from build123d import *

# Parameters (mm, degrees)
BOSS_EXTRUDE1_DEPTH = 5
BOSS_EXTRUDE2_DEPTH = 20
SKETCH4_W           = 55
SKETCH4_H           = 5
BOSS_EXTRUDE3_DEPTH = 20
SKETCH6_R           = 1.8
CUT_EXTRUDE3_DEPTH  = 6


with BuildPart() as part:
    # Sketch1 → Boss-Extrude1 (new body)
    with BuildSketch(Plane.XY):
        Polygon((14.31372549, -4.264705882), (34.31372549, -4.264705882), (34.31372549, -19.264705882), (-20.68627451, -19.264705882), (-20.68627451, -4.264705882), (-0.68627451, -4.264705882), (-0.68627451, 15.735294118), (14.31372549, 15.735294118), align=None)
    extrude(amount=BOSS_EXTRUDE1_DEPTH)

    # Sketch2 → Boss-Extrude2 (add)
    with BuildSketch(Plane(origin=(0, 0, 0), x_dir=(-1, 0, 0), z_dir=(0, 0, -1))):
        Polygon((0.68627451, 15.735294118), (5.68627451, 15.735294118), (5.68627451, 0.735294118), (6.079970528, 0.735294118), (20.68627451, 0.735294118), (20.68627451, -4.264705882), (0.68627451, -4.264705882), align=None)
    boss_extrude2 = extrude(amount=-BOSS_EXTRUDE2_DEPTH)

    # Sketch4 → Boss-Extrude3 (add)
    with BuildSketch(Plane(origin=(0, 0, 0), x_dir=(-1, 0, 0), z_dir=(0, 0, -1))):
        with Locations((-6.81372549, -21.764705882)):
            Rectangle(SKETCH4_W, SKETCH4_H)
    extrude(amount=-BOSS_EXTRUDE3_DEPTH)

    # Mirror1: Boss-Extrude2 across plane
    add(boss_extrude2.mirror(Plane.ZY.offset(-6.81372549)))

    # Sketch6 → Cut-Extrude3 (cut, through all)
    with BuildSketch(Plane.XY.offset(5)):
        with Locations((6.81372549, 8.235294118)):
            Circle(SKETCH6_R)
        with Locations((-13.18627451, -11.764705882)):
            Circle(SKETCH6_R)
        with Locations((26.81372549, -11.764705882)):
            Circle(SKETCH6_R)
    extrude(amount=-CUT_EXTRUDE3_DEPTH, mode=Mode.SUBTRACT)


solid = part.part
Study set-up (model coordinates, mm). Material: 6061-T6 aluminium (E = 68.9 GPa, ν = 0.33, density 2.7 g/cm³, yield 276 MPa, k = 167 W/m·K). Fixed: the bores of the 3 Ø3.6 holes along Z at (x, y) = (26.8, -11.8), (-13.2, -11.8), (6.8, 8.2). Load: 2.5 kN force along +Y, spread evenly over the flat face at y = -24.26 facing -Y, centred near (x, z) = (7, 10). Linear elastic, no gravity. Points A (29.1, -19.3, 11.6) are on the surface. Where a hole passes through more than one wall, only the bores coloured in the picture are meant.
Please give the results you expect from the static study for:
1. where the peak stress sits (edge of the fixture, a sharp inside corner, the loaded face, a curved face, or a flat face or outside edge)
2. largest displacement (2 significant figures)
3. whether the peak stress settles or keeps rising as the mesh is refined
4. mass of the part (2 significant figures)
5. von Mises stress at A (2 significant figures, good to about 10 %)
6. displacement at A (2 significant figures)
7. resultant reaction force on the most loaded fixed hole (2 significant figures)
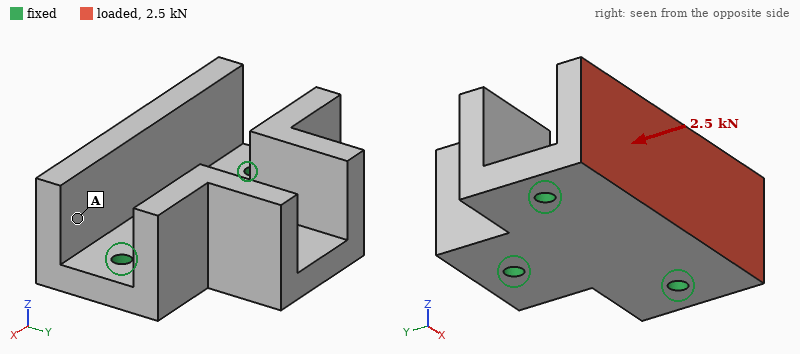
edge of the fixture
0.12 mm
keeps rising
49 g
17 MPa
0.056 mm
900 N
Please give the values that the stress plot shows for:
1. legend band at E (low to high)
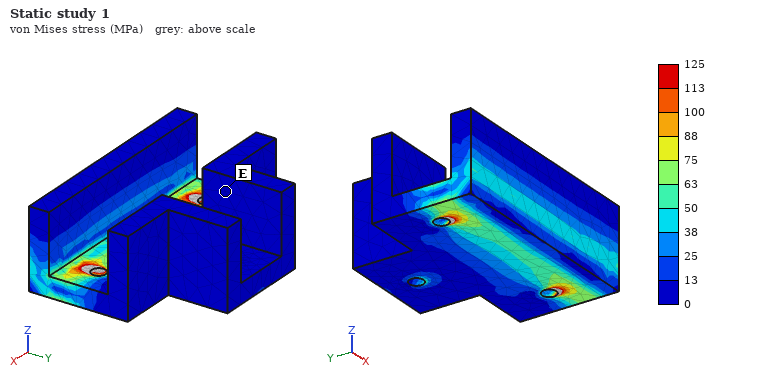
0 to 13 MPa
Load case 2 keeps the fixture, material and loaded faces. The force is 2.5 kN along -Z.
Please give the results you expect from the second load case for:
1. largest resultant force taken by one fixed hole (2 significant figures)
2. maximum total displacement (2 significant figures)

1.4 kN
0.13 mm
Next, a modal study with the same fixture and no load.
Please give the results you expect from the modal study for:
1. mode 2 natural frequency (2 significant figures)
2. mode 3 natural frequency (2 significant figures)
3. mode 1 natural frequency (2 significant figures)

9400 Hz
9500 Hz
6400 Hz
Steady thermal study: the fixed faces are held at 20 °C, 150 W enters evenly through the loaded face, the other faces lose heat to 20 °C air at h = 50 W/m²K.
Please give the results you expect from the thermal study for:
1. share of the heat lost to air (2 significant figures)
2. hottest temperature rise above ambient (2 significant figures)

4.8 %
65 K
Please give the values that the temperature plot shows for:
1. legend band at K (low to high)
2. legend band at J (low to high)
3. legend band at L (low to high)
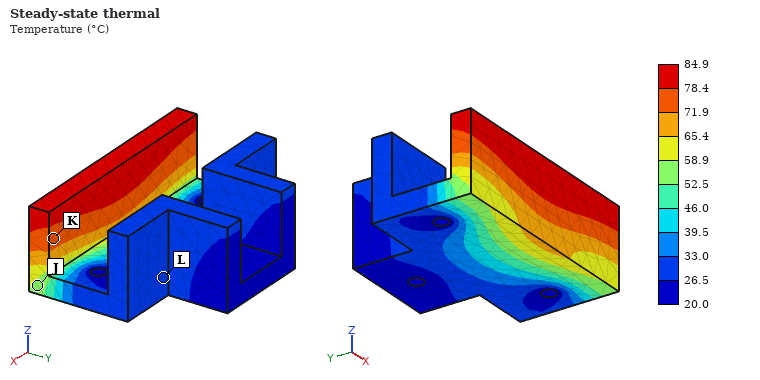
71.9 to 78.4 °C
52.5 to 58.9 °C
26.5 to 33.0 °C
